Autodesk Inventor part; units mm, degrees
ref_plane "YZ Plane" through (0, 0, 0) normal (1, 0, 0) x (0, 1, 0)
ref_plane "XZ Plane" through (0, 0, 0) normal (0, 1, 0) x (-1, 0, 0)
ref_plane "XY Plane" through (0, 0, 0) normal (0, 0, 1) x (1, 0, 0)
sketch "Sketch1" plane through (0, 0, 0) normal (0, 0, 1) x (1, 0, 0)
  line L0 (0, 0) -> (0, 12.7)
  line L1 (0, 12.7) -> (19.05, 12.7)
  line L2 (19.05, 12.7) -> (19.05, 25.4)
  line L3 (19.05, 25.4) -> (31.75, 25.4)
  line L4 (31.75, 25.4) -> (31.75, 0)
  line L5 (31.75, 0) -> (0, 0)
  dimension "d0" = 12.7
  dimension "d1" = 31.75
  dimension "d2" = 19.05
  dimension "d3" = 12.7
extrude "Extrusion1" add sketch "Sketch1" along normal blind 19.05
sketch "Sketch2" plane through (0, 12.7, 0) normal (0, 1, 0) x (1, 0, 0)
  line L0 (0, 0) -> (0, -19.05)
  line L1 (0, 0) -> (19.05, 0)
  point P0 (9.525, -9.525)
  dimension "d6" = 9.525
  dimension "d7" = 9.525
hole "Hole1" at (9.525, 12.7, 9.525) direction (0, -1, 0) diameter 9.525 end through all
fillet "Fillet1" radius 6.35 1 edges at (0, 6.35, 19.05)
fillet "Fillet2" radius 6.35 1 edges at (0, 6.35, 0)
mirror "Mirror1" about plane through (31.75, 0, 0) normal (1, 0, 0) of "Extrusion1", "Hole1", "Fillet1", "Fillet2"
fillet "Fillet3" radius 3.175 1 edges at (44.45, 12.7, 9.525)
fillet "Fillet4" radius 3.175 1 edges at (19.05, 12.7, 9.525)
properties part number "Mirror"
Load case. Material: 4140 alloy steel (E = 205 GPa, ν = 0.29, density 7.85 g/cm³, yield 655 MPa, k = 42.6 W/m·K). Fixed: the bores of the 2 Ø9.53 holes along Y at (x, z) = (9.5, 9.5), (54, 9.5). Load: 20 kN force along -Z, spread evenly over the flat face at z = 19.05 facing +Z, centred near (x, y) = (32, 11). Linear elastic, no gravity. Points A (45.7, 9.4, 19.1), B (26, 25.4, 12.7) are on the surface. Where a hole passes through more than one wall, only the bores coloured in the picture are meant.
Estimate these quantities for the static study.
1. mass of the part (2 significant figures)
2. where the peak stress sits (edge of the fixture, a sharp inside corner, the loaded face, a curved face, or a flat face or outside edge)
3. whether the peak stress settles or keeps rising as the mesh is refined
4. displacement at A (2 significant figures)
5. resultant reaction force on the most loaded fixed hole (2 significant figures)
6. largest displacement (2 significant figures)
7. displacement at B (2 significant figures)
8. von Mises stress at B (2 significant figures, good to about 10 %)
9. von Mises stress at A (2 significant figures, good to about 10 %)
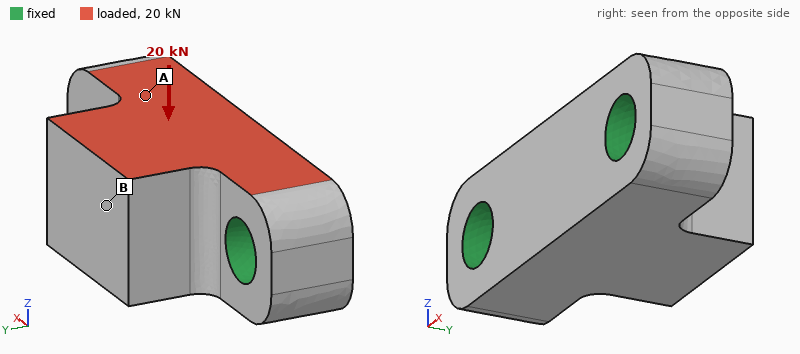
150 g
edge of the fixture
keeps rising
6.9 µm
10 kN
22 µm
20 µm
19 MPa
94 MPa
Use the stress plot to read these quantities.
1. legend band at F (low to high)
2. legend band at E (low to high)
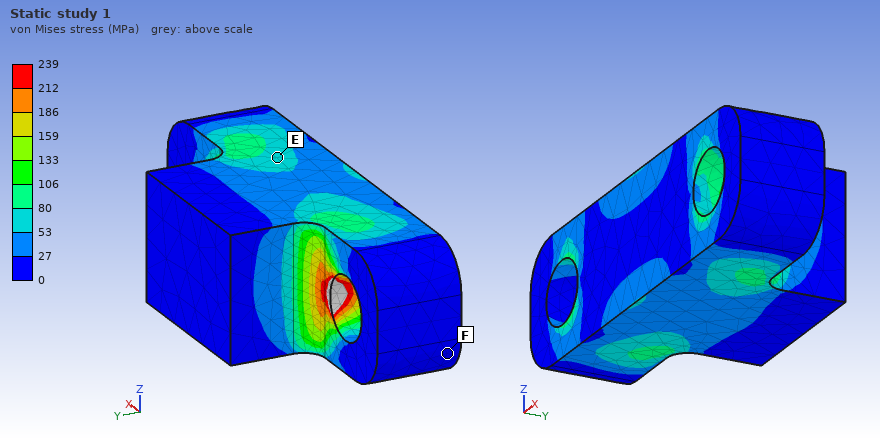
0 to 27 MPa
53 to 80 MPa
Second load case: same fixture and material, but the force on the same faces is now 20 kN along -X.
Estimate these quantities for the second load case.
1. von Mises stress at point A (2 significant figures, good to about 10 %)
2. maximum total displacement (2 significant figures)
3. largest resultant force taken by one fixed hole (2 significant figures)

48 MPa
10 µm
11 kN
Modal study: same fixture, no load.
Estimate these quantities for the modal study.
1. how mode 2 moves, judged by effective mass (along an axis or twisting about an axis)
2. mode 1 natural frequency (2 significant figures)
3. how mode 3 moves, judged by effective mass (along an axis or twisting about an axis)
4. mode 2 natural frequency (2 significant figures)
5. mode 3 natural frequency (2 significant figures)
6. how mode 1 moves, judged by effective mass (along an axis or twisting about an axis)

along Y
15 kHz
along Z
25 kHz
31 kHz
along Z
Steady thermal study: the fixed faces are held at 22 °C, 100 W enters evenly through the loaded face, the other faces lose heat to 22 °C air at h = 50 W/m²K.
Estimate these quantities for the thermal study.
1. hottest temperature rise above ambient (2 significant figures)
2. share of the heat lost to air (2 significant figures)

63 K
4.5 %
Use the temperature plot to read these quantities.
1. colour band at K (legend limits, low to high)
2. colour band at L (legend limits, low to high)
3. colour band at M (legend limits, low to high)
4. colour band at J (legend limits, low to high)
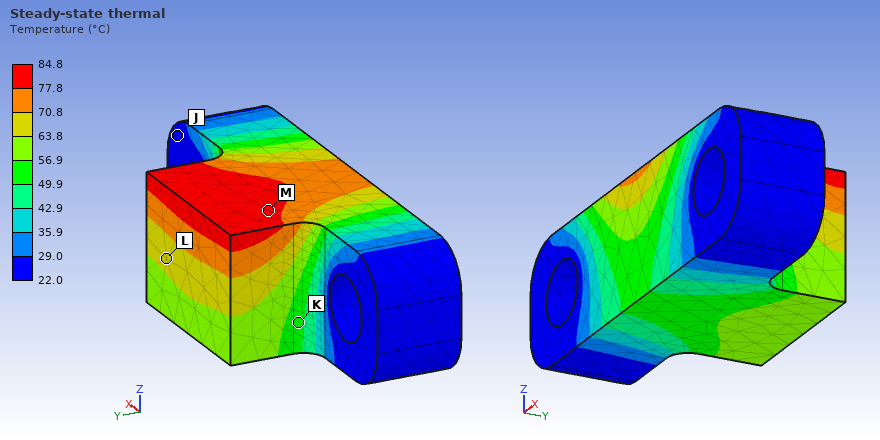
49.9 to 56.9 °C
63.8 to 70.8 °C
77.8 to 84.8 °C
22.0 to 29.0 °C
